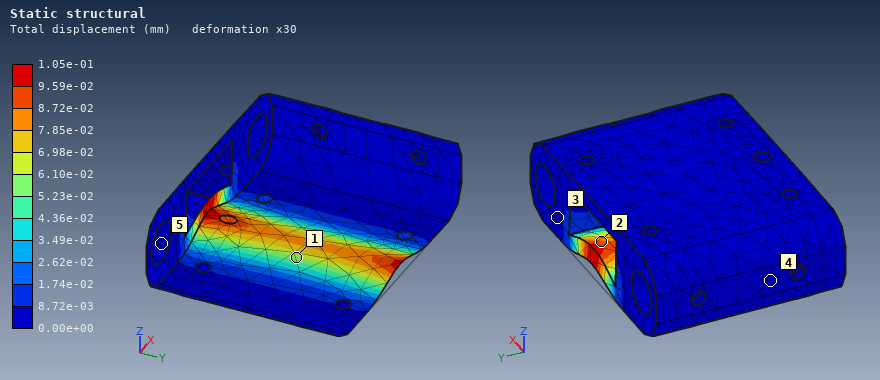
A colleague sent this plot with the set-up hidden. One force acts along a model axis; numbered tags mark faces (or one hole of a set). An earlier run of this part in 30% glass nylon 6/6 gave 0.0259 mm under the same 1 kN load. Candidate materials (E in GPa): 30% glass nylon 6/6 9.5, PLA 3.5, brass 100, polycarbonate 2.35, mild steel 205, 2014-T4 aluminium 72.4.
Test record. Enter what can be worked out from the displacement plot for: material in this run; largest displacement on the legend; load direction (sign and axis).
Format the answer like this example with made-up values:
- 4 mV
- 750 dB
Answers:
- polycarbonate
- 1.05e-01 mm
- +Z
